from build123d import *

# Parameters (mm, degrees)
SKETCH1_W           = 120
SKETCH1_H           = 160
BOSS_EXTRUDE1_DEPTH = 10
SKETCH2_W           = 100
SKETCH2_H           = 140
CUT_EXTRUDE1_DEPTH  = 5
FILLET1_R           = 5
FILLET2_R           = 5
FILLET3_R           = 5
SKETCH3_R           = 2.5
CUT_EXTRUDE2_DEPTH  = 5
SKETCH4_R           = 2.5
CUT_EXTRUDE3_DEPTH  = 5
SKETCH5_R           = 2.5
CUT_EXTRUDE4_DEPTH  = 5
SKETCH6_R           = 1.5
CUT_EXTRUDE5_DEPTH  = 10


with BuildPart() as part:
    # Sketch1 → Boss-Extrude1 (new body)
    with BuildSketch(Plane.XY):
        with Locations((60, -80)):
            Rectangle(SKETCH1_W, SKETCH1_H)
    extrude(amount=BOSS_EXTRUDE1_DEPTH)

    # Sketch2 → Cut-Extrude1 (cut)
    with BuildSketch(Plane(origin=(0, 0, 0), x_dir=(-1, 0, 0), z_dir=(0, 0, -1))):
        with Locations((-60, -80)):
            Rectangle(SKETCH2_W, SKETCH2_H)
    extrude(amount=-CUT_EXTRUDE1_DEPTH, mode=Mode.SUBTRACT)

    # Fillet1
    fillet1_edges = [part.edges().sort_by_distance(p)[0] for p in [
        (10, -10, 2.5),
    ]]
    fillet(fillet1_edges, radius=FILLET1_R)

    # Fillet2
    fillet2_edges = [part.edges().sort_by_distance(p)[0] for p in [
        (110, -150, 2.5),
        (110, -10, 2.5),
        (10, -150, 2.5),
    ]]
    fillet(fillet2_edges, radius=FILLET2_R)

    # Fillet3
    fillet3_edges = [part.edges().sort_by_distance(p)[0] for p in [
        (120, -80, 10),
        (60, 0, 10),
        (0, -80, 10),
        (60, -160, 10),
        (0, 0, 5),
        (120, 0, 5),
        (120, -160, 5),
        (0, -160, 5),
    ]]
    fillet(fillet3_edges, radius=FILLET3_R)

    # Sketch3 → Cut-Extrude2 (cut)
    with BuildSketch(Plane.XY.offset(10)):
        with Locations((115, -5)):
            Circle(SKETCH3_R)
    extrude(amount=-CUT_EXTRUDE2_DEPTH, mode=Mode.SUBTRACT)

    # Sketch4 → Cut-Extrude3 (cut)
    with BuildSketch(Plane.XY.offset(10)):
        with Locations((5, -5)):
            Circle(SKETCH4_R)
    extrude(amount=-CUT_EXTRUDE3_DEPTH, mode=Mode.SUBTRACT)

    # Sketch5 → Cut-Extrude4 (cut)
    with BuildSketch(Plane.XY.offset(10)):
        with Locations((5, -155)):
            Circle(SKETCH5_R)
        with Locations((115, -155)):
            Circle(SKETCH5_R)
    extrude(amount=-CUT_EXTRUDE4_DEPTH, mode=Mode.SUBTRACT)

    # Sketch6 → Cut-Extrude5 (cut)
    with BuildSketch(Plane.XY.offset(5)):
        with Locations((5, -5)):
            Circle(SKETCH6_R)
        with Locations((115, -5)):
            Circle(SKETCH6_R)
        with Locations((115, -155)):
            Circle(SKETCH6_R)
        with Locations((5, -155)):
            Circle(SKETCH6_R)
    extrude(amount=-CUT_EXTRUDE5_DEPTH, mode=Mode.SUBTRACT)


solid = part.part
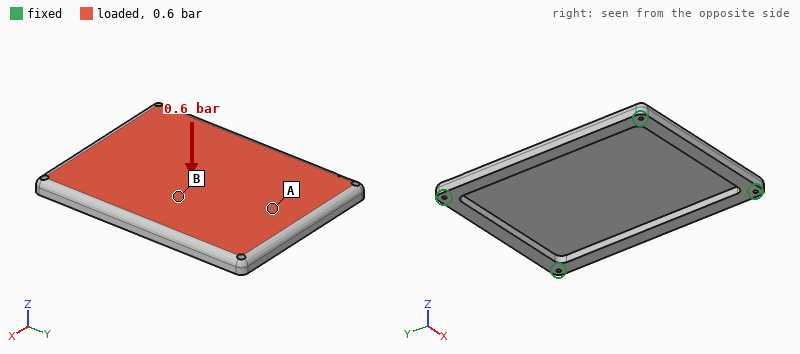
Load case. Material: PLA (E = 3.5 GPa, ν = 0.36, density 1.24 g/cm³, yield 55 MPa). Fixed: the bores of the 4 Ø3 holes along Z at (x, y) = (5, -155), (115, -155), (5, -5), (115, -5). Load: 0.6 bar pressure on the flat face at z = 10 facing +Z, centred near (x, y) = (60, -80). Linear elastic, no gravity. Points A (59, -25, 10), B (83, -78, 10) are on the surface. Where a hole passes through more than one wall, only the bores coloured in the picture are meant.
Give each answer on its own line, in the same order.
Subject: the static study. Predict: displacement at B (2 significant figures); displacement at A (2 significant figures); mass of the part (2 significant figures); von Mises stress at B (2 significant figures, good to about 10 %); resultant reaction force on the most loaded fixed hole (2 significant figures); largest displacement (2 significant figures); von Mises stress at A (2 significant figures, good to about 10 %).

1.7 mm
0.92 mm
150 g
11 MPa
750 N
1.9 mm
6.2 MPa
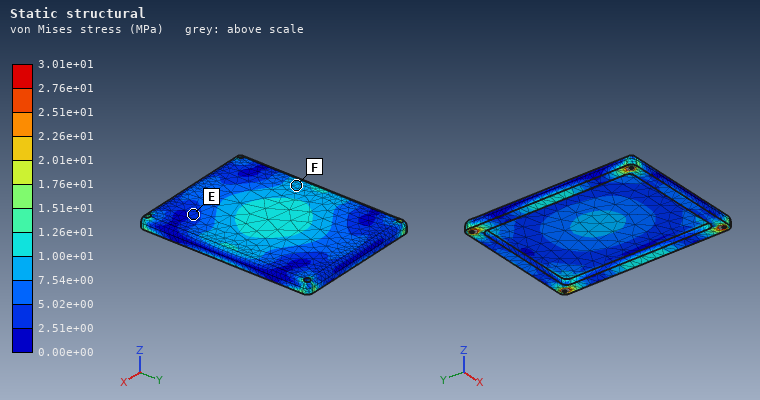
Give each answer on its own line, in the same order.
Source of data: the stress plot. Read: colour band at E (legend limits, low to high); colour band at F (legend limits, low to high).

2.51e+00 to 5.02e+00 MPa
7.54e+00 to 1.00e+01 MPa
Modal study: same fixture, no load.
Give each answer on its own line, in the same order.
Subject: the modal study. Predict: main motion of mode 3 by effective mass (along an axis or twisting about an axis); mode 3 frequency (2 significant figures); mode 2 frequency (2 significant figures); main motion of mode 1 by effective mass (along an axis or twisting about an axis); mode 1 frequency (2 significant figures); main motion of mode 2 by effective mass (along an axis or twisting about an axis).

twisting about X
840 Hz
610 Hz
along Z
410 Hz
twisting about Y
